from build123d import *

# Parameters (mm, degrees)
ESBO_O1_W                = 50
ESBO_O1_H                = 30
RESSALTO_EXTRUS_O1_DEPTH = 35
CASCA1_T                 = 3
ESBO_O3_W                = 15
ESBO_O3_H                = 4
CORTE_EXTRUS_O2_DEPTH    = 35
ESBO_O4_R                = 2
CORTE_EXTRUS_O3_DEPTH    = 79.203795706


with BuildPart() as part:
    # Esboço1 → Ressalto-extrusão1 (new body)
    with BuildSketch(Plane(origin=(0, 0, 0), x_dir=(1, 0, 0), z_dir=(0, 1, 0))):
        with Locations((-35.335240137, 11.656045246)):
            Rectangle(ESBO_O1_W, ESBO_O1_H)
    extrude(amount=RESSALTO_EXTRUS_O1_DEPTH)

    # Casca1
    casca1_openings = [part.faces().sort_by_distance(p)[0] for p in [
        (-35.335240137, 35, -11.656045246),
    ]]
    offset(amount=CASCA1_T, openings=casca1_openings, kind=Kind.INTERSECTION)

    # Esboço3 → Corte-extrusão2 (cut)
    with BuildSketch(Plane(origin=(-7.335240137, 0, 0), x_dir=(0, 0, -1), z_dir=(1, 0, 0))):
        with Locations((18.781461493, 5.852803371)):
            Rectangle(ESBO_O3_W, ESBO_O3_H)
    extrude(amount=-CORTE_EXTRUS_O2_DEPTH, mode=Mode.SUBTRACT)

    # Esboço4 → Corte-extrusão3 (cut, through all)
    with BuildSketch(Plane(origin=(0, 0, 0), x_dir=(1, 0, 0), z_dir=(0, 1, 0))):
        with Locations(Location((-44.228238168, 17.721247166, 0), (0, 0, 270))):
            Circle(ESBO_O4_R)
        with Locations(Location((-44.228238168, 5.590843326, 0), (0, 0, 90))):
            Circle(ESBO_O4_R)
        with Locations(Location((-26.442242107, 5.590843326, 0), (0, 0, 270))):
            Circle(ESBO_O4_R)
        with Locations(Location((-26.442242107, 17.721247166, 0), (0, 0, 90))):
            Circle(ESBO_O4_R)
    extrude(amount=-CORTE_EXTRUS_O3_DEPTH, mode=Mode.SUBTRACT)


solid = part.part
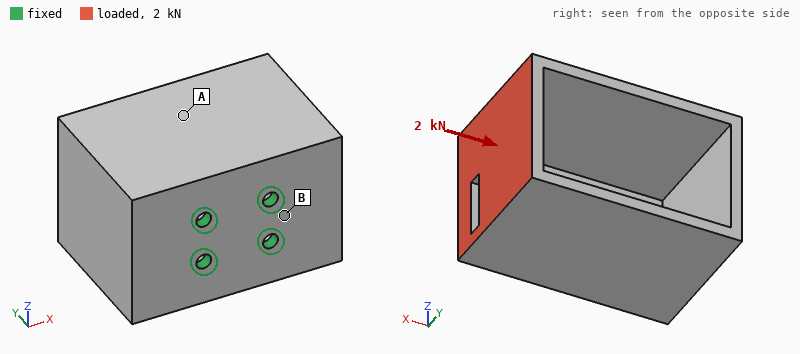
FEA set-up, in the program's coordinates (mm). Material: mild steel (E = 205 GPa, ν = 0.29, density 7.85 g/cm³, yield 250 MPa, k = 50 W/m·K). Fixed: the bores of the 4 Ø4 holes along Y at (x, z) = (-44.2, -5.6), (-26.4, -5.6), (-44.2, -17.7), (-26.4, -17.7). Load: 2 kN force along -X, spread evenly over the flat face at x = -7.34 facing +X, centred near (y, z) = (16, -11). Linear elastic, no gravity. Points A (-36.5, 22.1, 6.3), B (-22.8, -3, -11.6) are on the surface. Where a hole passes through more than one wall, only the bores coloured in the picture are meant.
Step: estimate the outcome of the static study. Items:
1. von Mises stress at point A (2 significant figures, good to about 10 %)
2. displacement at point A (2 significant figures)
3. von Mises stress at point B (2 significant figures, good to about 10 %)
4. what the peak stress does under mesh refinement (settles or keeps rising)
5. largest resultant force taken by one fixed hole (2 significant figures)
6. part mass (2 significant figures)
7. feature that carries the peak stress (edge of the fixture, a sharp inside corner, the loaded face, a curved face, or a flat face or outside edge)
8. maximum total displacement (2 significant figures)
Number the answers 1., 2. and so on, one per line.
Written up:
1. 15 MPa
2. 28 µm
3. 56 MPa
4. keeps rising
5. 970 N
6. 190 g
7. edge of the fixture
8. 73 µm
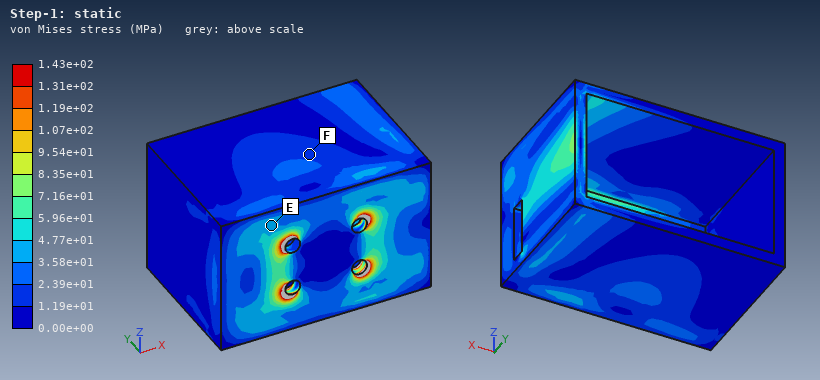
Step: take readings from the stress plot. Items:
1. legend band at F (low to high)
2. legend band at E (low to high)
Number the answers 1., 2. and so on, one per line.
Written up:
1. 1.19e+01 to 2.39e+01 MPa
2. 3.58e+01 to 4.77e+01 MPa
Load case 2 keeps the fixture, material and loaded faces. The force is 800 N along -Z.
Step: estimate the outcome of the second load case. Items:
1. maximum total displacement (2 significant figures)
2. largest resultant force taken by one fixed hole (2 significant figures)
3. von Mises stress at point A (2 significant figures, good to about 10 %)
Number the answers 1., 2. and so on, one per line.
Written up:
1. 46 µm
2. 870 N
3. 12 MPa
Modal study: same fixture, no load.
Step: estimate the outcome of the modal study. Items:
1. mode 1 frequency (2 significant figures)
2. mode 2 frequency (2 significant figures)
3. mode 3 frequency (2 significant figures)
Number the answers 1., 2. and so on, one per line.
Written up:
1. 2500 Hz
2. 2600 Hz
3. 2900 Hz
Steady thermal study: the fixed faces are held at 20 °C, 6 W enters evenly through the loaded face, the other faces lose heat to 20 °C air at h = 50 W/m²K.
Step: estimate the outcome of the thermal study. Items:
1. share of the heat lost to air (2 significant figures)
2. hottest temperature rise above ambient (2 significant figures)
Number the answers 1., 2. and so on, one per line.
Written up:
1. 46 %
2. 13 K
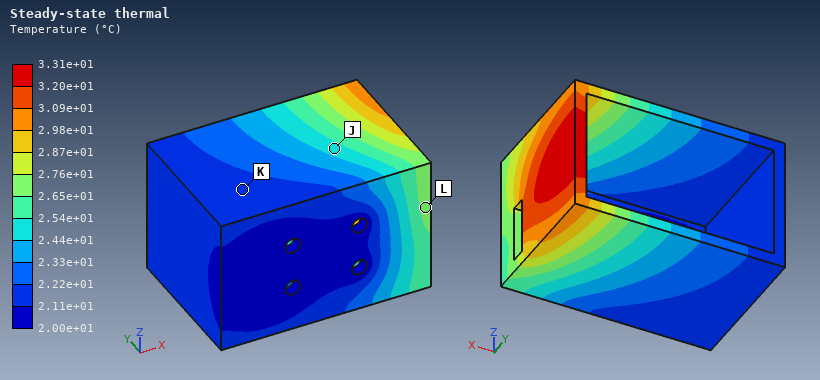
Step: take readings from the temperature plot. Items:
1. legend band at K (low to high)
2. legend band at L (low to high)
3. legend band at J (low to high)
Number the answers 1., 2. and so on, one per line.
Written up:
1. 2.11e+01 to 2.22e+01 °C
2. 2.65e+01 to 2.76e+01 °C
3. 2.44e+01 to 2.54e+01 °C
